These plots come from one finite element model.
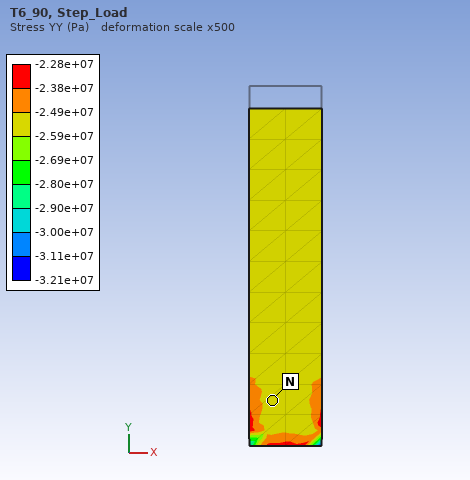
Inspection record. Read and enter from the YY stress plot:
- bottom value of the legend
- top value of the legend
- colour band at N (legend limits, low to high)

-3.21e+07 Pa
-2.28e+07 Pa
-2.59e+07 to -2.49e+07 Pa
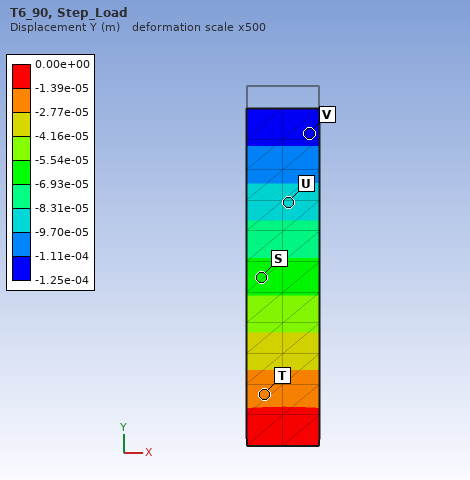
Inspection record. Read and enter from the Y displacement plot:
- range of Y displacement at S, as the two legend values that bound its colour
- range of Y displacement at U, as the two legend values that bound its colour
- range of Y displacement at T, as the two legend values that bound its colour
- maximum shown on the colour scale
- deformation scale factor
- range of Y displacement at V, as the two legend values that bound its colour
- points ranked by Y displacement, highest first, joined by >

-6.93e-05 to -5.54e-05 m
-9.70e-05 to -8.31e-05 m
-2.77e-05 to -1.39e-05 m
0.00e+00 m
500
-1.25e-04 to -1.11e-04 m
T > S > U > V
